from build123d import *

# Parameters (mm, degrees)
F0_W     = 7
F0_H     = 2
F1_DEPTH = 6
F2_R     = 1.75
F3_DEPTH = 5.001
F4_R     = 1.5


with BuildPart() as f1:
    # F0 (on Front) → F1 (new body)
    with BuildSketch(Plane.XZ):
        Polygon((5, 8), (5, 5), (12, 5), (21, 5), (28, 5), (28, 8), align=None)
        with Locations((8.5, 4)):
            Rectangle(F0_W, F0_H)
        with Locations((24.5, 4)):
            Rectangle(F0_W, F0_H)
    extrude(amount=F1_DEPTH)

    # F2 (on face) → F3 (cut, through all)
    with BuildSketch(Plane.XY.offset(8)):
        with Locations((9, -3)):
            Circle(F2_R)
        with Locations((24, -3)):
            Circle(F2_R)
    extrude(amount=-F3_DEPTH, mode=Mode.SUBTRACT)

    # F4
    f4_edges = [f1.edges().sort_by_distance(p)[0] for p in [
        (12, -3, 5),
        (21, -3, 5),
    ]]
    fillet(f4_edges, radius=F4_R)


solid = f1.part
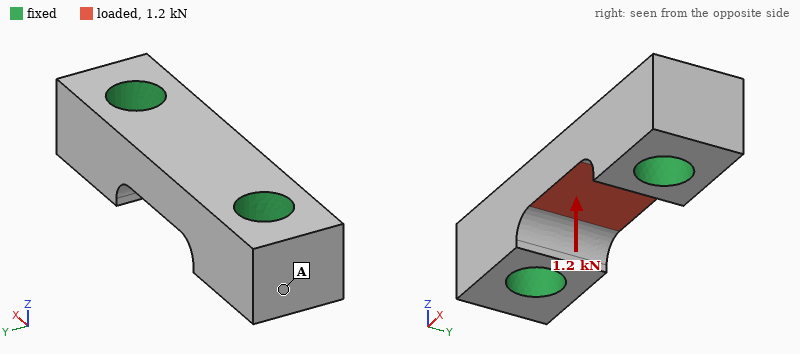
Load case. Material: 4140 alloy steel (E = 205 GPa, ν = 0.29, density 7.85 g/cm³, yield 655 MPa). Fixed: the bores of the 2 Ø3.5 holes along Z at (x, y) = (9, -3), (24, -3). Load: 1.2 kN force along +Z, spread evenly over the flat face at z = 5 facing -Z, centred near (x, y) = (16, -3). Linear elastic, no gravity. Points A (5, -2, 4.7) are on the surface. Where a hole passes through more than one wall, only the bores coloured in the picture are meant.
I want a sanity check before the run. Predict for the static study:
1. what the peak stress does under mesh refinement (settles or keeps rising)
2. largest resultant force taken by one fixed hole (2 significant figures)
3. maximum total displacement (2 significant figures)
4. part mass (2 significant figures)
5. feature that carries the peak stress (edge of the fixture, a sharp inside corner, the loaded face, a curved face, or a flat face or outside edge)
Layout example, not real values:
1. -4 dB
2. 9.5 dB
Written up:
1. keeps rising
2. 610 N
3. 4.1 µm
4. 3.9 g
5. edge of the fixture
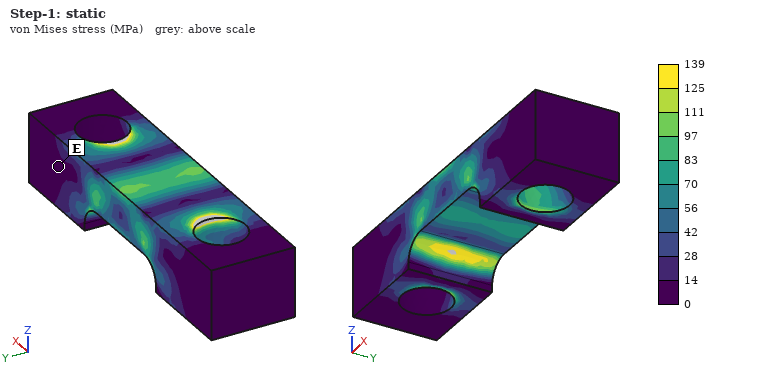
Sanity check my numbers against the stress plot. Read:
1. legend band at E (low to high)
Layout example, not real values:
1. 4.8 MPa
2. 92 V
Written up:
1. 0 to 14 MPa
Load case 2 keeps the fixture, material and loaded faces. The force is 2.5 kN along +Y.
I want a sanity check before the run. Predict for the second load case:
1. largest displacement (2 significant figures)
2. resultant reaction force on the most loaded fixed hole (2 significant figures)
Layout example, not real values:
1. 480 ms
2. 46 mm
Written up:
1. 12 µm
2. 1.3 kN
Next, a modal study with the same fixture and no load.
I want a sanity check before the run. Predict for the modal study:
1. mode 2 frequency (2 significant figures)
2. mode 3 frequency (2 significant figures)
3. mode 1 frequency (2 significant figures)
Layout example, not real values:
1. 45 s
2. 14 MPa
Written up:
1. 100 kHz
2. 130 kHz
3. 98 kHz
